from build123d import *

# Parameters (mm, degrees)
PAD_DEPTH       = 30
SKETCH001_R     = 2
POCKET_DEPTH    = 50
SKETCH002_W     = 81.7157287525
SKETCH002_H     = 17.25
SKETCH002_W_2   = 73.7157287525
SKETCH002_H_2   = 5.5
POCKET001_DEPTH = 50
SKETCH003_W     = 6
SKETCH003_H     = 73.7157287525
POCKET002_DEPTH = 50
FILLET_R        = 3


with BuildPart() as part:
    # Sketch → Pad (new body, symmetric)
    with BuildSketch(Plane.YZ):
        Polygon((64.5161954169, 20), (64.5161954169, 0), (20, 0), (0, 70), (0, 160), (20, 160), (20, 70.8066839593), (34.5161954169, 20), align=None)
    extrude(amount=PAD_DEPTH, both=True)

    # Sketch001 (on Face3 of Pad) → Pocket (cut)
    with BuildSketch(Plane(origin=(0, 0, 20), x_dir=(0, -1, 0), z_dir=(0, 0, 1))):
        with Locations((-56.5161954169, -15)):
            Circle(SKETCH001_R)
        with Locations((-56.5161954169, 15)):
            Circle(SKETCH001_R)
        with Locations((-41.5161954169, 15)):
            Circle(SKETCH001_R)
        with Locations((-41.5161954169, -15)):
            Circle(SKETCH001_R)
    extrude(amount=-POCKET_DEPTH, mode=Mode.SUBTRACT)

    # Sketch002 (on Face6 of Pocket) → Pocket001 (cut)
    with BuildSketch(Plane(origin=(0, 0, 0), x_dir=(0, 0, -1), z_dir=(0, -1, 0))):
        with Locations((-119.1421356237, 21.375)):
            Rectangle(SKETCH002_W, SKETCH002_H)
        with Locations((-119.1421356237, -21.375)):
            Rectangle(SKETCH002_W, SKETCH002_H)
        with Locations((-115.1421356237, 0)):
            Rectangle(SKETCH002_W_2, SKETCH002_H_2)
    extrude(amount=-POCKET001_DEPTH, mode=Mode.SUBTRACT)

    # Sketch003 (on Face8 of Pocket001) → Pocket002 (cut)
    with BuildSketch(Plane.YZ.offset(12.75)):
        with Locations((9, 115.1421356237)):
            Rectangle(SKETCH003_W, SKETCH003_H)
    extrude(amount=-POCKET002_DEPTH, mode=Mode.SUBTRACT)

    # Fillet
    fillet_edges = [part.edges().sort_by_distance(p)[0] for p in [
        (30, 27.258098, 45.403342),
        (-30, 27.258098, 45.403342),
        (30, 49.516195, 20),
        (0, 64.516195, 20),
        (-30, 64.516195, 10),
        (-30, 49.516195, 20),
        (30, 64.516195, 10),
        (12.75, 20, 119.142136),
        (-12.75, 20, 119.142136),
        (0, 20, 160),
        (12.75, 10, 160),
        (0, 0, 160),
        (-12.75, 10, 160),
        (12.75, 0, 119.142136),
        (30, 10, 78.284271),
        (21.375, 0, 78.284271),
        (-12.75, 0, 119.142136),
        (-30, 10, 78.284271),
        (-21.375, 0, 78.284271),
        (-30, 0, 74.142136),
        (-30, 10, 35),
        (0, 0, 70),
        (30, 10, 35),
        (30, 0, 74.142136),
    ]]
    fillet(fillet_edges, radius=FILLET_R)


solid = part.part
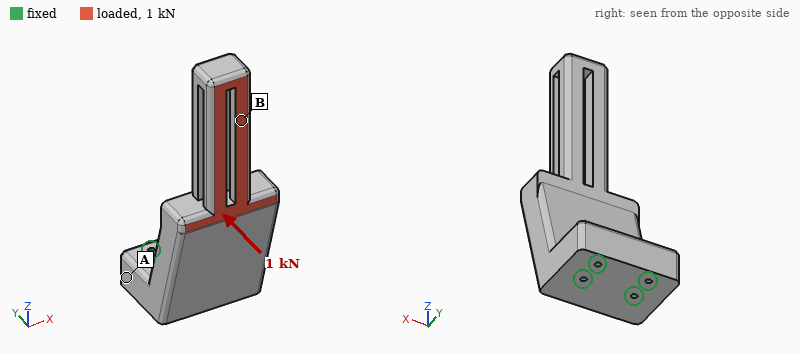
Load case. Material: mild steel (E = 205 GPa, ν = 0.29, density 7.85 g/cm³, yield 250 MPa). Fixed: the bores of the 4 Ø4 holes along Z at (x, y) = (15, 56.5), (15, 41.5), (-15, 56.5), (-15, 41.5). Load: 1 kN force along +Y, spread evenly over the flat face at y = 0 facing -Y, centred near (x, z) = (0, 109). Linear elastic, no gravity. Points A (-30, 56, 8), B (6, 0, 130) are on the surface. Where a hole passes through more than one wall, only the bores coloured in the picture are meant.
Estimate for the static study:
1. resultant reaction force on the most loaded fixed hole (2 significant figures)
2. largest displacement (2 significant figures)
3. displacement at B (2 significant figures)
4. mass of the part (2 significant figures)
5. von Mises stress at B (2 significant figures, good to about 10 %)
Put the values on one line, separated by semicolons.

960 N; 0.20 mm; 0.16 mm; 1.2 kg; 22 MPa
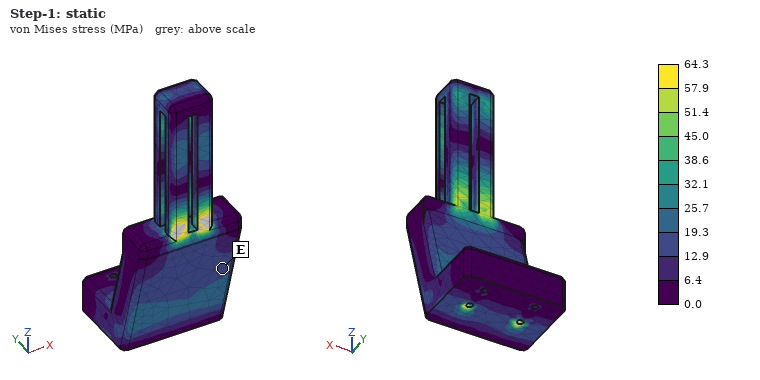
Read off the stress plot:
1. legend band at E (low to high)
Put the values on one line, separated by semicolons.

12.9 to 19.3 MPa
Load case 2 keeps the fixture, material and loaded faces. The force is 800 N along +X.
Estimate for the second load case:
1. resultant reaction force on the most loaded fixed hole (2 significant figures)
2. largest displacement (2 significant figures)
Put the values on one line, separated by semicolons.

1.9 kN; 68 µm
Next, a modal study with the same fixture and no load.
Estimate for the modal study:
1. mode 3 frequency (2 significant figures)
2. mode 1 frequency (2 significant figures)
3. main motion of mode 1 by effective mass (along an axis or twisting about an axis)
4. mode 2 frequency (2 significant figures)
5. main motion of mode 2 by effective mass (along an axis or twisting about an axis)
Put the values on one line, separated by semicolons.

2500 Hz; 820 Hz; along Y; 1300 Hz; along X
